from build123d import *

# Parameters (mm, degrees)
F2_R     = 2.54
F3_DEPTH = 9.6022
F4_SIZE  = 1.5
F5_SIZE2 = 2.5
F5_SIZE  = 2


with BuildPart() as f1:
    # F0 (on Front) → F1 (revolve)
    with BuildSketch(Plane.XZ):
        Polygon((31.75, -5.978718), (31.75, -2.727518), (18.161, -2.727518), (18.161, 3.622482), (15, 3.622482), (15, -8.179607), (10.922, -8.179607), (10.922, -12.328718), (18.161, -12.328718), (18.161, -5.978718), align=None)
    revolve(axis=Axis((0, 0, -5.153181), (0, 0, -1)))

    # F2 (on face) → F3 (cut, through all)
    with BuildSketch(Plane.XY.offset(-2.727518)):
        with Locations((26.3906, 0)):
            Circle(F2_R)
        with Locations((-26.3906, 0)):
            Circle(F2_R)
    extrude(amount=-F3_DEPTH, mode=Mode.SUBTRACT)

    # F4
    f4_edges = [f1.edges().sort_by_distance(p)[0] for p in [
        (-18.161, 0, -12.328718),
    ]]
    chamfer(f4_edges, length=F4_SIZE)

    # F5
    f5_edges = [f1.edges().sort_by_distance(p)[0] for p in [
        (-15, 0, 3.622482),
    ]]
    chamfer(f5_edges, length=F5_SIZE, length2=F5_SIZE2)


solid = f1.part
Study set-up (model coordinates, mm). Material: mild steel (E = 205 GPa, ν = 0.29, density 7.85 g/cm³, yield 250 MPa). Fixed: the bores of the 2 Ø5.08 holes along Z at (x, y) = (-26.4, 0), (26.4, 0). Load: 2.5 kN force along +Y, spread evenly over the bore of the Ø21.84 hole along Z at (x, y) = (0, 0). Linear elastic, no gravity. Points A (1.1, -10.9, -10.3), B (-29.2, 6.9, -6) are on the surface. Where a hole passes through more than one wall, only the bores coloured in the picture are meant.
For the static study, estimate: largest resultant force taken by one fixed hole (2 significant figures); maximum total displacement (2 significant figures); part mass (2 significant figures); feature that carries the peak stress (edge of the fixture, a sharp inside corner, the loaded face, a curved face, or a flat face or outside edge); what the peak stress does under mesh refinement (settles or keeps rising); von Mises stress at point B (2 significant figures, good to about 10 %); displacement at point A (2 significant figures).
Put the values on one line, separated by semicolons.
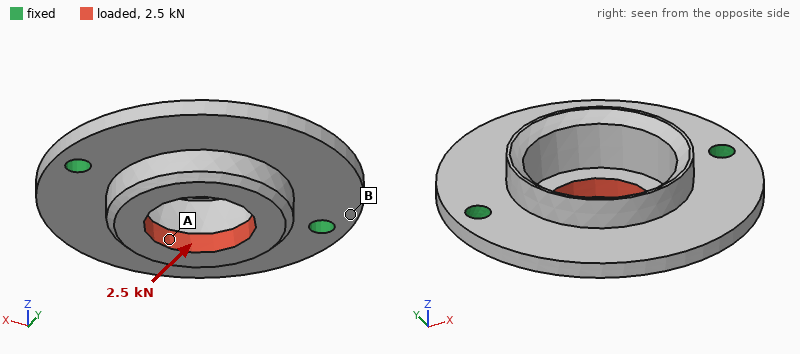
1.3 kN; 73 µm; 100 g; edge of the fixture; keeps rising; 82 MPa; 28 µm
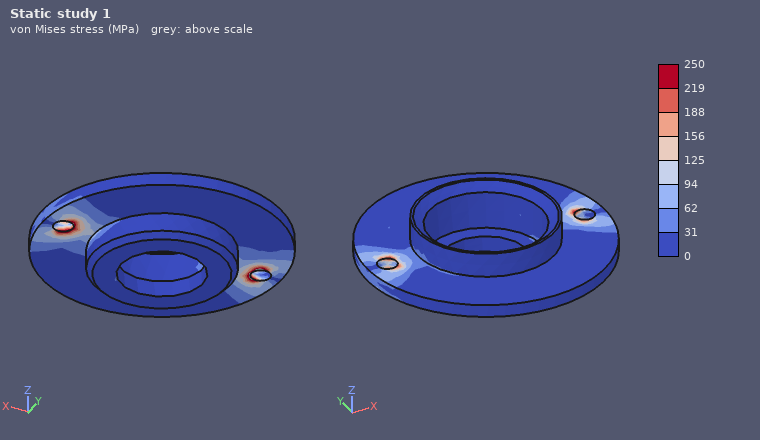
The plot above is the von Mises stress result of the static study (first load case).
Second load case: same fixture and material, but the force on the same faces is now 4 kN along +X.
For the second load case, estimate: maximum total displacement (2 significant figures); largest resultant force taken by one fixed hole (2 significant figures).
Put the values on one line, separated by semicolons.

6.8 µm; 2.1 kN
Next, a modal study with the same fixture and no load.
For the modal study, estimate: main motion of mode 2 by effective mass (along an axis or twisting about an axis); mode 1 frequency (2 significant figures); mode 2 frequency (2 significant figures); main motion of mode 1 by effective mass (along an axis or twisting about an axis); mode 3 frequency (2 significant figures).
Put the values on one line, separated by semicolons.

along Z; 2600 Hz; 5000 Hz; twisting about X; 9300 Hz
